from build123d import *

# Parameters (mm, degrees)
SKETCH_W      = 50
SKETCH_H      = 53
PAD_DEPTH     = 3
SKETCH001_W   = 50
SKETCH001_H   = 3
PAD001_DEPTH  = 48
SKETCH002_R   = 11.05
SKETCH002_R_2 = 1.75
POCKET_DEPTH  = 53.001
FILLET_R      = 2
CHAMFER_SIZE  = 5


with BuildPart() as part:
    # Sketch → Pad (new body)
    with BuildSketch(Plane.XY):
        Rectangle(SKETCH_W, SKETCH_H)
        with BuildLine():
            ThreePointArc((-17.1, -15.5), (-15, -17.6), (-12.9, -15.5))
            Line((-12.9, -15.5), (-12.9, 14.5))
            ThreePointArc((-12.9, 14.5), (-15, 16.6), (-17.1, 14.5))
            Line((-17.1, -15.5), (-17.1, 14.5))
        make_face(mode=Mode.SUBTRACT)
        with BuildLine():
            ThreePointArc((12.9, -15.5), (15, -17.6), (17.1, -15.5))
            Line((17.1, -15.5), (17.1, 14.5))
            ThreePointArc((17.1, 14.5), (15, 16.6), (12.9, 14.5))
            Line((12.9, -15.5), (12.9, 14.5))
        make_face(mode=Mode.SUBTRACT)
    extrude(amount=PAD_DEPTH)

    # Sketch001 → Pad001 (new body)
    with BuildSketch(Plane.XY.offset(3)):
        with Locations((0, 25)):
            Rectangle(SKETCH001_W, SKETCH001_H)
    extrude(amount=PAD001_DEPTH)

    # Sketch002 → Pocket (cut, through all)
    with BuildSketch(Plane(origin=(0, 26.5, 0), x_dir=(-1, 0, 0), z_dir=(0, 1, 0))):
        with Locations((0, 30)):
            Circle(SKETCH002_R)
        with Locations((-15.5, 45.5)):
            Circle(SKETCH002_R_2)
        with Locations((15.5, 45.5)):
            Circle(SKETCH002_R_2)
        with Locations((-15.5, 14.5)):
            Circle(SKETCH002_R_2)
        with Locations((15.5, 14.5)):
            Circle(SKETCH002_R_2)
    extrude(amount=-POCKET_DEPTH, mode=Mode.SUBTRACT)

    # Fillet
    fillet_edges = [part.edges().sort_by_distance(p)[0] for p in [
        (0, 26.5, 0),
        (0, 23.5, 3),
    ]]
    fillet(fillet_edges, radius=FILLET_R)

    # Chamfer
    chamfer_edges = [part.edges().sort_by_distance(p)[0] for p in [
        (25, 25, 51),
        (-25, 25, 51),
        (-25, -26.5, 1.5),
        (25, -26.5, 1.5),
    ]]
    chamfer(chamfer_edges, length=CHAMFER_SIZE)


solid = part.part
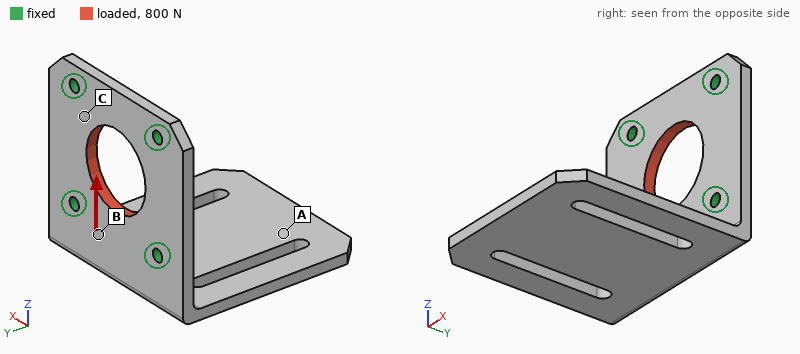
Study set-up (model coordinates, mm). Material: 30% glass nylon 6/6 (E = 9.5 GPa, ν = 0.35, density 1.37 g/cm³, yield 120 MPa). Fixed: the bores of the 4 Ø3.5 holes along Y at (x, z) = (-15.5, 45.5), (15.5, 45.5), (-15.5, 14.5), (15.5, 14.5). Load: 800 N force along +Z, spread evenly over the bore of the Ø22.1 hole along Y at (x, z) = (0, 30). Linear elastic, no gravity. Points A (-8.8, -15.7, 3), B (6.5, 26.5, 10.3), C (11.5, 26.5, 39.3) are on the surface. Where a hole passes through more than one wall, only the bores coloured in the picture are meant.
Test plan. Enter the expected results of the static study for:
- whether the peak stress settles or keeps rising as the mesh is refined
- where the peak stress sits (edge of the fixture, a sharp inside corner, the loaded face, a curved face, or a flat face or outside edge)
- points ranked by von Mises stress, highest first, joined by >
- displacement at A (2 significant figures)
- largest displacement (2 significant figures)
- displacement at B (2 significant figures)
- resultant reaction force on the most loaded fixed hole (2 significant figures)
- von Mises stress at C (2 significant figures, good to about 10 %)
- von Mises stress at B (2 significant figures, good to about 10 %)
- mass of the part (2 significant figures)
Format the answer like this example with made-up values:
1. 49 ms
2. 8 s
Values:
1. keeps rising
2. edge of the fixture
3. C > B > A
4. 6.4 µm
5. 18 µm
6. 6.1 µm
7. 210 N
8. 5.7 MPa
9. 2.8 MPa
10. 18 g
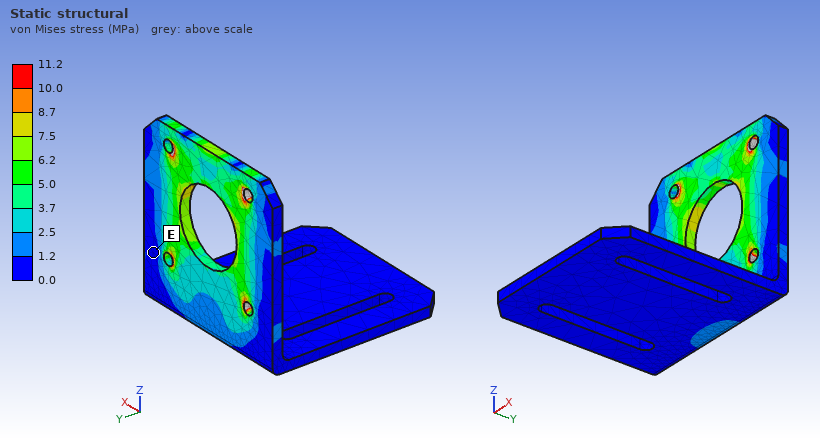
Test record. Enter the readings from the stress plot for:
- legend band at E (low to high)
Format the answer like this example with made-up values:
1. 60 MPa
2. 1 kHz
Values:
1. 0.0 to 1.2 MPa
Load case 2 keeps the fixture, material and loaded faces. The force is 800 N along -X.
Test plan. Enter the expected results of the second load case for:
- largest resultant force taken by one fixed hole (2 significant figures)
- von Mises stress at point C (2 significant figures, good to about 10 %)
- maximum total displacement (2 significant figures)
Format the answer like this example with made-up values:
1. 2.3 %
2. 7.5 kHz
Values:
1. 210 N
2. 4.4 MPa
3. 14 µm
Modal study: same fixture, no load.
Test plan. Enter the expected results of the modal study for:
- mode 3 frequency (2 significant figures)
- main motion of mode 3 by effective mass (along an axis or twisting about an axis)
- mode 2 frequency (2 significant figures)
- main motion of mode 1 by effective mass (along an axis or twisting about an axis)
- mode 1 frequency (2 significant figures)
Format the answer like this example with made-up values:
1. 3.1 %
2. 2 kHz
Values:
1. 1400 Hz
2. along X
3. 970 Hz
4. along Z
5. 370 Hz
